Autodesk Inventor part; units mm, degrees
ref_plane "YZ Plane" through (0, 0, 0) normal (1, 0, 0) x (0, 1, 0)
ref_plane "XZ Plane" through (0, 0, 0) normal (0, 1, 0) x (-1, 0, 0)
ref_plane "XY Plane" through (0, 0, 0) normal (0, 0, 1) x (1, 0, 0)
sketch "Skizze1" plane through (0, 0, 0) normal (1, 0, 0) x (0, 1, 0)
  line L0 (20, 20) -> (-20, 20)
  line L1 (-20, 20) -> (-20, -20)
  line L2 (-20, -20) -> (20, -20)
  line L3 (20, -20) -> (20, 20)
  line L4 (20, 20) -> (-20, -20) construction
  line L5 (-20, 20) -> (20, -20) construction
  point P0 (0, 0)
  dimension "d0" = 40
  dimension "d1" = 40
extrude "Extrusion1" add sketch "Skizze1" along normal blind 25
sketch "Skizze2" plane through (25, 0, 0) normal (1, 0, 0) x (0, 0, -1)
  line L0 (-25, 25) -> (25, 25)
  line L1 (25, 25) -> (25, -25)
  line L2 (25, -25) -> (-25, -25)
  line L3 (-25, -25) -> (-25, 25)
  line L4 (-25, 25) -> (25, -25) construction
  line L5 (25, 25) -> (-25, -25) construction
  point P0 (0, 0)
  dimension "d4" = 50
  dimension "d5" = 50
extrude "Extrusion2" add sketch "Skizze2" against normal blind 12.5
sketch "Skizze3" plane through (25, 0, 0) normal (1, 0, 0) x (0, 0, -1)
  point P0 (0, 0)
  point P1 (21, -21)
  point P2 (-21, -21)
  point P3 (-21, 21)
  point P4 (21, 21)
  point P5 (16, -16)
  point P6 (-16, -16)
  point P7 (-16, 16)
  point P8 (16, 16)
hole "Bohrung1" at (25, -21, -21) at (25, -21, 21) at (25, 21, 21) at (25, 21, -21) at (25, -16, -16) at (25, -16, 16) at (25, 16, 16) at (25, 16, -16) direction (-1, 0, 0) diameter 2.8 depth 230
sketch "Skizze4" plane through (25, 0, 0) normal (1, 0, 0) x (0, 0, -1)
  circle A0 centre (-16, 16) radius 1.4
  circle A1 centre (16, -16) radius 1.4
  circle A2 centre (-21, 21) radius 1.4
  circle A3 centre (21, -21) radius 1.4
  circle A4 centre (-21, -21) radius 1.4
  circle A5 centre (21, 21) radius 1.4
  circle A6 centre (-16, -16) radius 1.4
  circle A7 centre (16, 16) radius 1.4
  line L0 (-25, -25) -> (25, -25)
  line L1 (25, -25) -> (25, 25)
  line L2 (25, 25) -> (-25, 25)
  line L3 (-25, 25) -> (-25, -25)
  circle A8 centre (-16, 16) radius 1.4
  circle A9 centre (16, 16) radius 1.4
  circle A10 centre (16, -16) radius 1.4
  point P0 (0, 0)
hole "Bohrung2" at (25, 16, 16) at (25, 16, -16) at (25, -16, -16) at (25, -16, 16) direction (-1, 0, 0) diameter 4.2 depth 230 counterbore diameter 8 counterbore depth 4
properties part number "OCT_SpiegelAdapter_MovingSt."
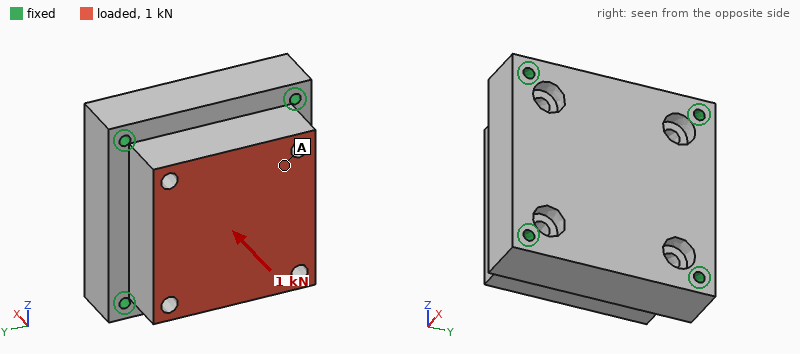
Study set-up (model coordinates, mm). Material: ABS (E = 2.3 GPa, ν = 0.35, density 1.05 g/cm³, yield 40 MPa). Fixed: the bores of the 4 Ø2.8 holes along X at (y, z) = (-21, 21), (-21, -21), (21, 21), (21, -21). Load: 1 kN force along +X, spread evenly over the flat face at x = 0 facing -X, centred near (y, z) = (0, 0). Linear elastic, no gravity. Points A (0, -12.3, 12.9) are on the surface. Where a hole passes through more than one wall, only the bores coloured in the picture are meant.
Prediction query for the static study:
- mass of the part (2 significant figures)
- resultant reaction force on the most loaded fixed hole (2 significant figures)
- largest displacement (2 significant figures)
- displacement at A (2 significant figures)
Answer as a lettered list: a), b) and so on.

a) 51 g
b) 260 N
c) 33 µm
d) 29 µm
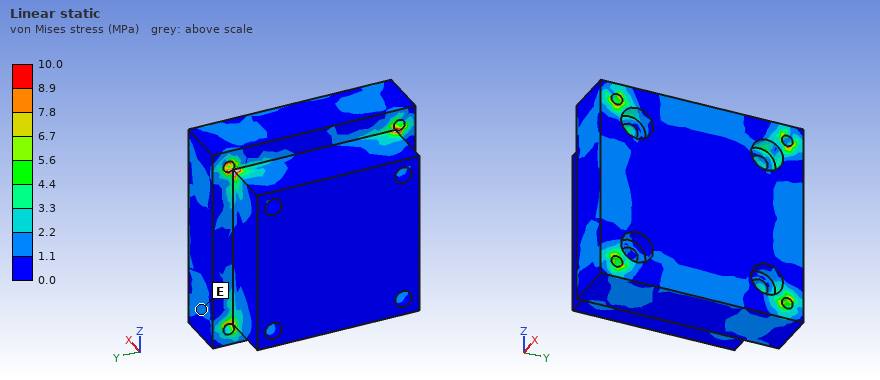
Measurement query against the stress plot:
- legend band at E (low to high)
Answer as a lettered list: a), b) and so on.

a) 1.1 to 2.2 MPa
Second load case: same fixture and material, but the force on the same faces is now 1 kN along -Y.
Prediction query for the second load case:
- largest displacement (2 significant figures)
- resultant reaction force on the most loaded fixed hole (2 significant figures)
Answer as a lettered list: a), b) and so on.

a) 56 µm
b) 350 N
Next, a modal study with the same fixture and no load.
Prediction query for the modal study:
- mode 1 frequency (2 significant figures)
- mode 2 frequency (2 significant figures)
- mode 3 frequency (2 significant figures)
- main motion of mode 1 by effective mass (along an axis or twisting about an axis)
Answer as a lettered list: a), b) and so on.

a) 4400 Hz
b) 5300 Hz
c) 5300 Hz
d) along X
